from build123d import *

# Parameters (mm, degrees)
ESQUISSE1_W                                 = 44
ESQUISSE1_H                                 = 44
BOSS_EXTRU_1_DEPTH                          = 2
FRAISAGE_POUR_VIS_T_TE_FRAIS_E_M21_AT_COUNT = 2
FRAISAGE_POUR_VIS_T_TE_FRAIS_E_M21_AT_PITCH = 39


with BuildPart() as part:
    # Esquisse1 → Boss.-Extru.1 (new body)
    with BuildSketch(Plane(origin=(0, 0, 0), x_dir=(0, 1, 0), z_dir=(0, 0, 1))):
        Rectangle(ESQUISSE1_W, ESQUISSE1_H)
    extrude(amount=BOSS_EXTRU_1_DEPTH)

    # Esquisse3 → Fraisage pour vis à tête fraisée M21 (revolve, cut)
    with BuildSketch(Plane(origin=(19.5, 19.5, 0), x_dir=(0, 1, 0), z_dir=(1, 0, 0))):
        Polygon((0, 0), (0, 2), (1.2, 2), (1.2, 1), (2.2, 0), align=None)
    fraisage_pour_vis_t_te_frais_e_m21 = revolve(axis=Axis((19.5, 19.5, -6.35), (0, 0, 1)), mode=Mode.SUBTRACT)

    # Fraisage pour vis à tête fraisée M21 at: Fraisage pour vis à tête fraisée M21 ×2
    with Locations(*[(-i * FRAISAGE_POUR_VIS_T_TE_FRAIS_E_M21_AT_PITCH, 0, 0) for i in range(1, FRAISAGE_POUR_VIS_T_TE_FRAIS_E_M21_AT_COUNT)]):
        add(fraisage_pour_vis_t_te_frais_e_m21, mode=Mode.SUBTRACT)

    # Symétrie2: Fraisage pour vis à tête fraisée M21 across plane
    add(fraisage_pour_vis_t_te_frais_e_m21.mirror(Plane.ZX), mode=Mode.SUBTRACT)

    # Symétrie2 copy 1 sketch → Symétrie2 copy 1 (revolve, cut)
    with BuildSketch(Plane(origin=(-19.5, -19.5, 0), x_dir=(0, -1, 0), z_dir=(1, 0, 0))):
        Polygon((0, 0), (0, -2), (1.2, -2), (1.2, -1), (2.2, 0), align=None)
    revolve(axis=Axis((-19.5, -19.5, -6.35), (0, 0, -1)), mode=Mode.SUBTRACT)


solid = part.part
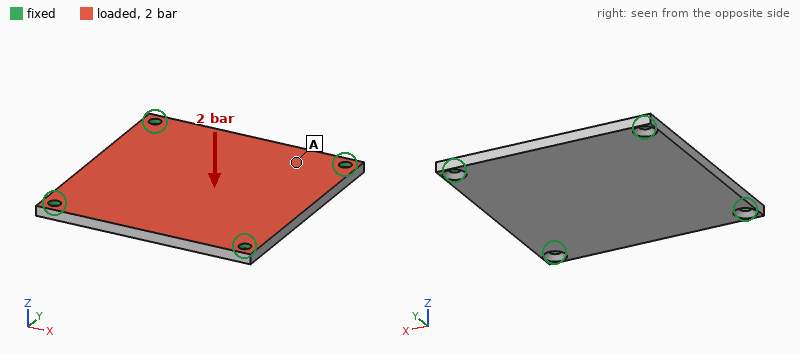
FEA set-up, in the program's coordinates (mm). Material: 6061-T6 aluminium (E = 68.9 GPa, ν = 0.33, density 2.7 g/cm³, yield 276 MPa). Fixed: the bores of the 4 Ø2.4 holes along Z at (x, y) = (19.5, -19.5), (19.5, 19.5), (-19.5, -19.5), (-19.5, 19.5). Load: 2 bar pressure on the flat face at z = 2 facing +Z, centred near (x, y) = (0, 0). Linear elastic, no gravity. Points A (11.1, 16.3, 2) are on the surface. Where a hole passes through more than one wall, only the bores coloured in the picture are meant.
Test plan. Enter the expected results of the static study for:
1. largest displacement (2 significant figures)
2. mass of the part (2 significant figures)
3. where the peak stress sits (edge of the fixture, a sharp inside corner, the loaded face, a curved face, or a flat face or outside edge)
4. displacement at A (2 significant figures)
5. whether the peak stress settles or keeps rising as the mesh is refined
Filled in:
90 µm
10 g
edge of the fixture
37 µm
keeps rising
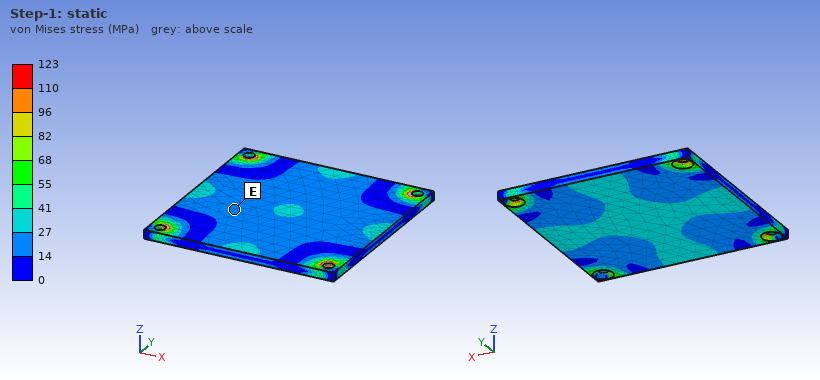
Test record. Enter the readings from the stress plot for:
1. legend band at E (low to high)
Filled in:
14 to 27 MPa
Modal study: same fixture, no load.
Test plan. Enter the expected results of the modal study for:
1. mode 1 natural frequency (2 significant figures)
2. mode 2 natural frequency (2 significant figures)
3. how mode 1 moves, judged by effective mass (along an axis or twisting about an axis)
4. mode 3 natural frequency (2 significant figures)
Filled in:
3900 Hz
6800 Hz
along Z
6800 Hz
